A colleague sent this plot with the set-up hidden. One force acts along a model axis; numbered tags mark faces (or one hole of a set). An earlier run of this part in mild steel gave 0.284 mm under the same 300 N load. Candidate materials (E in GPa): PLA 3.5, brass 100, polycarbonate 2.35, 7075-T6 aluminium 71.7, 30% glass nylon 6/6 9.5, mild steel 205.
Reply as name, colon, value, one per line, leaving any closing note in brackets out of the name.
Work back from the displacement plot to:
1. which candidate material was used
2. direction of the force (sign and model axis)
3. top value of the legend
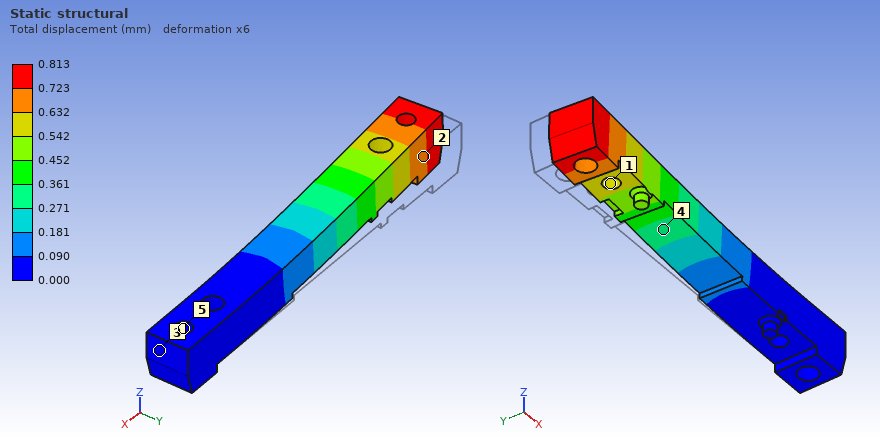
which candidate material was used: 7075-T6 aluminium
direction of the force: -Y
top value of the legend: 0.813 mm
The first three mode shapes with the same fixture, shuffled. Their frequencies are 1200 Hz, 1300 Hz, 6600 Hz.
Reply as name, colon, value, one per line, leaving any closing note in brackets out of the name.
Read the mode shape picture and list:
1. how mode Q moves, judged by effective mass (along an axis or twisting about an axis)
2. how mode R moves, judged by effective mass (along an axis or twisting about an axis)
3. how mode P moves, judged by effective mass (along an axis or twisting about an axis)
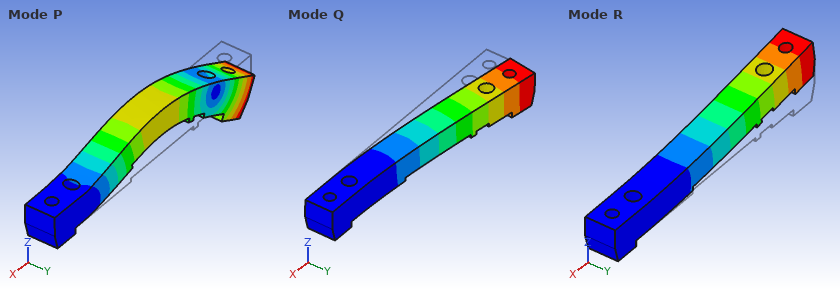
how mode Q moves, judged by effective mass: along Y
how mode R moves, judged by effective mass: along Z
how mode P moves, judged by effective mass: along Z
